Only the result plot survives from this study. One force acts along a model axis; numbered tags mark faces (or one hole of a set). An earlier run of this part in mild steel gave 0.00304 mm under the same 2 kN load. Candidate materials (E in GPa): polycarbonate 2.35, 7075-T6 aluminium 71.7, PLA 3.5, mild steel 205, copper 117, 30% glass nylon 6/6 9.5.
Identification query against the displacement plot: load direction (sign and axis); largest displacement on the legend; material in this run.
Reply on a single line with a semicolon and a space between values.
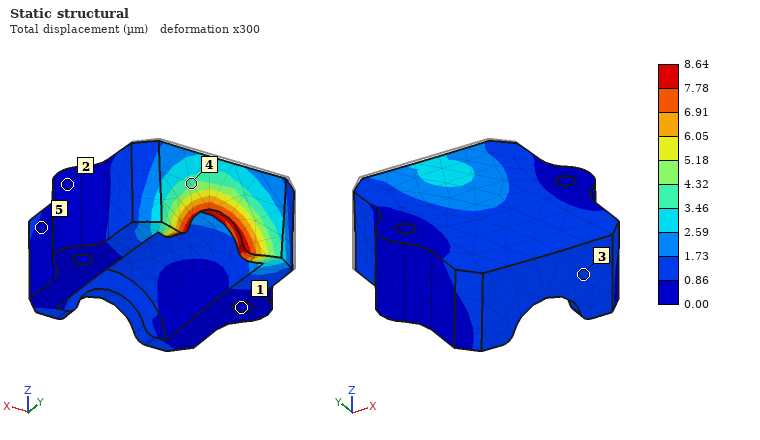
-Y; 8.64 µm; 7075-T6 aluminium
